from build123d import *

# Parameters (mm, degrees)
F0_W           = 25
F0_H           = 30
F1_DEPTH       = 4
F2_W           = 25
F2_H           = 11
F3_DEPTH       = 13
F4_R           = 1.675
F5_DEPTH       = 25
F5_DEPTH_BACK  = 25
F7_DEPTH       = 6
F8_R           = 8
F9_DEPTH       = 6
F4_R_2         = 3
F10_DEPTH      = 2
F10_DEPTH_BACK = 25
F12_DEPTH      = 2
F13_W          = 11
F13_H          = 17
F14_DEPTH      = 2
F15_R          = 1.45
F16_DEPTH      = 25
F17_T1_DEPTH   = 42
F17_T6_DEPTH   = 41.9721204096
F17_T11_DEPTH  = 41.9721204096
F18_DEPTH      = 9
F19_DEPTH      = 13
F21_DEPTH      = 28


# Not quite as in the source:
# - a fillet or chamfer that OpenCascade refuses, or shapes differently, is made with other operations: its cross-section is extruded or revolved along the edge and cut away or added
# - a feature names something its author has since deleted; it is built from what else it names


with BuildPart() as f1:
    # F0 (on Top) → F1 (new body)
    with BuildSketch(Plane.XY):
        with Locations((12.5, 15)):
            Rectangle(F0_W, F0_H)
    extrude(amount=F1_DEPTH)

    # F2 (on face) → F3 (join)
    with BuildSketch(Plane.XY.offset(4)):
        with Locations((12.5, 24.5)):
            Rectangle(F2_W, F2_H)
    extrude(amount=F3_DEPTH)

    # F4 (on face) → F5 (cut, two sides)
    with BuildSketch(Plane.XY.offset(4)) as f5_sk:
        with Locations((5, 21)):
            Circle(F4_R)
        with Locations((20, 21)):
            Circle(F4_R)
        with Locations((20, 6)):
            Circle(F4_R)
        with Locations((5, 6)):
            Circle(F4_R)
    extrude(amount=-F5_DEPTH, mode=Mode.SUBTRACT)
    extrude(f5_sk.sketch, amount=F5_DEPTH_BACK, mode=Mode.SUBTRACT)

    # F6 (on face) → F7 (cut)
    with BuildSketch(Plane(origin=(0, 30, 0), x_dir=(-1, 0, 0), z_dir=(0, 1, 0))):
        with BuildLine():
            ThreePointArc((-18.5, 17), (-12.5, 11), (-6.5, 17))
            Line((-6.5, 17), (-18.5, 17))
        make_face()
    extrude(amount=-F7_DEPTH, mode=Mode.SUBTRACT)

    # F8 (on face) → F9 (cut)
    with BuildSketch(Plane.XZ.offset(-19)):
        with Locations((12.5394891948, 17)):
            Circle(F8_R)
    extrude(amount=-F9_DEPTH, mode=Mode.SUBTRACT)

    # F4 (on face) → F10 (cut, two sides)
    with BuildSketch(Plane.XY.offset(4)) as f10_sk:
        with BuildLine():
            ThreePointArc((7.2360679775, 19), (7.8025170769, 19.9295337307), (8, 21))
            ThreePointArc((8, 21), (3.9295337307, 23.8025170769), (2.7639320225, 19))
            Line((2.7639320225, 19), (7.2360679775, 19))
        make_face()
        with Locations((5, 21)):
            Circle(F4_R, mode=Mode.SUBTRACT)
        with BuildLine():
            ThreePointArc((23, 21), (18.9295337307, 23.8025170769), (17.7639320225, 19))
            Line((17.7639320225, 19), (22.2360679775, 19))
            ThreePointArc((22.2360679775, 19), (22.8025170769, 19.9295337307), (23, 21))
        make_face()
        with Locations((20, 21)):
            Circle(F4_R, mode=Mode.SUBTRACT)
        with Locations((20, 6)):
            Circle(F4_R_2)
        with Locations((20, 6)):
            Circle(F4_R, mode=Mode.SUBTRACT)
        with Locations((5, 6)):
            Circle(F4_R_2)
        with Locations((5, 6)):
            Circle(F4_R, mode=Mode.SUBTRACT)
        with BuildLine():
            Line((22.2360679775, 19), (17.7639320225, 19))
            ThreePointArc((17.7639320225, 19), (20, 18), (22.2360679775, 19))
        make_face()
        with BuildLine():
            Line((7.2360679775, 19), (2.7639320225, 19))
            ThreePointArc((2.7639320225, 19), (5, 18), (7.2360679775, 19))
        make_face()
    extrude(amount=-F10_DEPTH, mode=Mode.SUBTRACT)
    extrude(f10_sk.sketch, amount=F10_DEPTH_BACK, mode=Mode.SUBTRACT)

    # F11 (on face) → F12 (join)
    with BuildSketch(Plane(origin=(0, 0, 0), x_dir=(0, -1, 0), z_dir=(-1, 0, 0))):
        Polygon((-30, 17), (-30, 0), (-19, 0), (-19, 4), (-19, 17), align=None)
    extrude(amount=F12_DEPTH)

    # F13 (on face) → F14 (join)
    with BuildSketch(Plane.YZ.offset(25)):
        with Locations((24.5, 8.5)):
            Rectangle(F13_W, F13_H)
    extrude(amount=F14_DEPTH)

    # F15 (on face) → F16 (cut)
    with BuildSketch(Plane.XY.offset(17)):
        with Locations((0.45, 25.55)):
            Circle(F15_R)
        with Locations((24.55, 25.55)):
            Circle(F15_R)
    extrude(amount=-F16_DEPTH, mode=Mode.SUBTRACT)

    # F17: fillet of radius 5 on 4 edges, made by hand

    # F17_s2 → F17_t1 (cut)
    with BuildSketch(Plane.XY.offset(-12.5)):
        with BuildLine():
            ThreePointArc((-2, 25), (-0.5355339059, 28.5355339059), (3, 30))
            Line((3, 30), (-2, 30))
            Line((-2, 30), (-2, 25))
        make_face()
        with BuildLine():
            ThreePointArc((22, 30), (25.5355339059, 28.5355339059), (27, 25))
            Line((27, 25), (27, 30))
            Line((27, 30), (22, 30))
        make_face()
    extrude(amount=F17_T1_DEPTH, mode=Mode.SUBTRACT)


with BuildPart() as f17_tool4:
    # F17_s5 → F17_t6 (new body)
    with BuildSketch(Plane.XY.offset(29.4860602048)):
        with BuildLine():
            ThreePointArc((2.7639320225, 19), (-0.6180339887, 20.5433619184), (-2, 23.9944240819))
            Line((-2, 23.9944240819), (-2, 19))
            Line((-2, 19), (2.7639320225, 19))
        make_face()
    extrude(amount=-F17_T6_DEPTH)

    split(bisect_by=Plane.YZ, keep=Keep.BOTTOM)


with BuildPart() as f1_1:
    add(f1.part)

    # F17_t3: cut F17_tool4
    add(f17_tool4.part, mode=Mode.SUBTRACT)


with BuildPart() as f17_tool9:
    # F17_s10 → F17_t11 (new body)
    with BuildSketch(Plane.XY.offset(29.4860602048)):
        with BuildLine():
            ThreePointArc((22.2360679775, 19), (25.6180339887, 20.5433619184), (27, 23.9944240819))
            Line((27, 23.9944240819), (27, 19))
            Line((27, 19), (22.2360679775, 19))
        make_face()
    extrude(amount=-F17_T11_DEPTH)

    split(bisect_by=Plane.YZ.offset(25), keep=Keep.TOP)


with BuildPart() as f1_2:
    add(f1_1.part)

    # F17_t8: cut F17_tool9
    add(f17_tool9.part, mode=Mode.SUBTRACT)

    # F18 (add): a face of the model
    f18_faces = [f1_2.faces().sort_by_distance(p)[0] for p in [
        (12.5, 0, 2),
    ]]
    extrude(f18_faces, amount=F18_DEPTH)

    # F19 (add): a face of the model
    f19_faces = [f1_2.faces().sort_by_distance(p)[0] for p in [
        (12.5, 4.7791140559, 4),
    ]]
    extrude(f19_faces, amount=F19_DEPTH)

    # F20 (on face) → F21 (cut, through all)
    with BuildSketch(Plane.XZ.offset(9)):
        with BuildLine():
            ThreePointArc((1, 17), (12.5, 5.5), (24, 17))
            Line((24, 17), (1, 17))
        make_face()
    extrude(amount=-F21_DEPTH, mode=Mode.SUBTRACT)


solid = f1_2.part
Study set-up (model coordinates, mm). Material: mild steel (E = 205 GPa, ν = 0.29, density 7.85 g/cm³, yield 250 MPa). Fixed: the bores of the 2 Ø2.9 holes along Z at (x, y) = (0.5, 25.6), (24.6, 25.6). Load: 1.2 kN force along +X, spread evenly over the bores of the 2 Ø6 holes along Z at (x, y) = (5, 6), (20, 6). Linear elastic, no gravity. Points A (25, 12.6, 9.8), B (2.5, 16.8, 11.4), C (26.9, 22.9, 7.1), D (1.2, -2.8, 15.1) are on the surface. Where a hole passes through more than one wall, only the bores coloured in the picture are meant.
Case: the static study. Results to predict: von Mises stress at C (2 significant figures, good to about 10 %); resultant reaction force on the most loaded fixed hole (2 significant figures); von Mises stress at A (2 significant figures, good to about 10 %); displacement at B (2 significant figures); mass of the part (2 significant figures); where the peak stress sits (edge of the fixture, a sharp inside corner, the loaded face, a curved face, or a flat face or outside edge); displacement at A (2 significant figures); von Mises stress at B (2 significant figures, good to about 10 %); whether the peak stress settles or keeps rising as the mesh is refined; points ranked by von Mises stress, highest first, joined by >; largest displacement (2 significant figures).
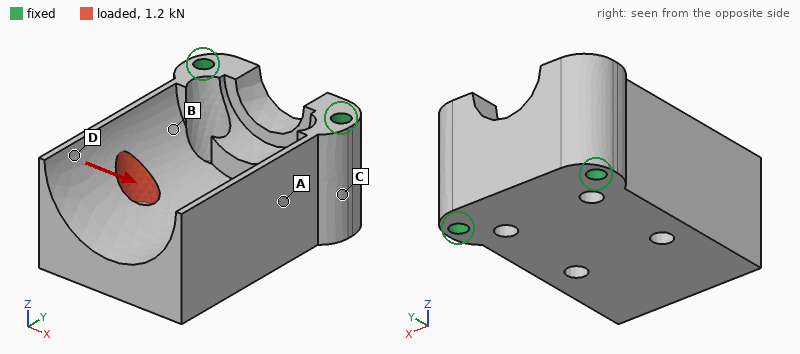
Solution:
14 MPa
1.1 kN
22 MPa
1.8 µm
70 g
edge of the fixture
3.6 µm
8.6 MPa
keeps rising
A > C > B > D
12 µm
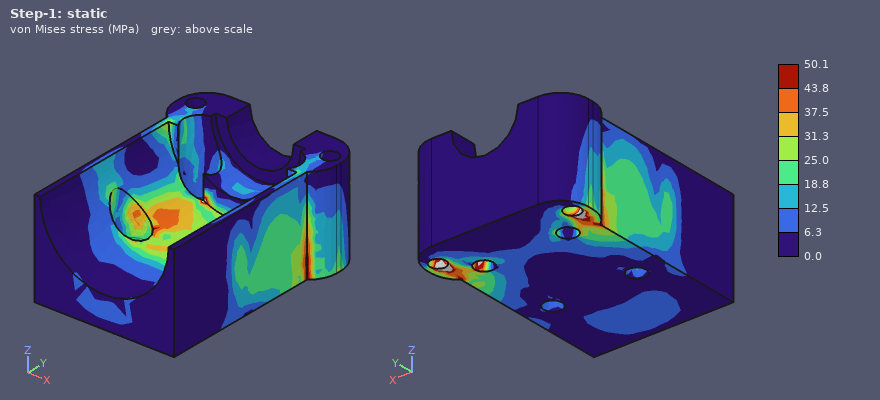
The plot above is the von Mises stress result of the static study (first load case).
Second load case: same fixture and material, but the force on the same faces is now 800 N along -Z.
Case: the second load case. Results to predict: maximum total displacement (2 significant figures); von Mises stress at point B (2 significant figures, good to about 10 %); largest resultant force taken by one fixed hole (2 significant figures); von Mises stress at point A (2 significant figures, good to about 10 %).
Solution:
9.0 µm
30 MPa
400 N
16 MPa
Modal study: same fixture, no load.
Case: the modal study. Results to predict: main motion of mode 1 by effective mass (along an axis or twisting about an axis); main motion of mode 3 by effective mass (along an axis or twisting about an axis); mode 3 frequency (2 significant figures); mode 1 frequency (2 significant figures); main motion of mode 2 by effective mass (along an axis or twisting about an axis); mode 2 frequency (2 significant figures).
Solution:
along Z
along X
16 kHz
7800 Hz
along X
9900 Hz
